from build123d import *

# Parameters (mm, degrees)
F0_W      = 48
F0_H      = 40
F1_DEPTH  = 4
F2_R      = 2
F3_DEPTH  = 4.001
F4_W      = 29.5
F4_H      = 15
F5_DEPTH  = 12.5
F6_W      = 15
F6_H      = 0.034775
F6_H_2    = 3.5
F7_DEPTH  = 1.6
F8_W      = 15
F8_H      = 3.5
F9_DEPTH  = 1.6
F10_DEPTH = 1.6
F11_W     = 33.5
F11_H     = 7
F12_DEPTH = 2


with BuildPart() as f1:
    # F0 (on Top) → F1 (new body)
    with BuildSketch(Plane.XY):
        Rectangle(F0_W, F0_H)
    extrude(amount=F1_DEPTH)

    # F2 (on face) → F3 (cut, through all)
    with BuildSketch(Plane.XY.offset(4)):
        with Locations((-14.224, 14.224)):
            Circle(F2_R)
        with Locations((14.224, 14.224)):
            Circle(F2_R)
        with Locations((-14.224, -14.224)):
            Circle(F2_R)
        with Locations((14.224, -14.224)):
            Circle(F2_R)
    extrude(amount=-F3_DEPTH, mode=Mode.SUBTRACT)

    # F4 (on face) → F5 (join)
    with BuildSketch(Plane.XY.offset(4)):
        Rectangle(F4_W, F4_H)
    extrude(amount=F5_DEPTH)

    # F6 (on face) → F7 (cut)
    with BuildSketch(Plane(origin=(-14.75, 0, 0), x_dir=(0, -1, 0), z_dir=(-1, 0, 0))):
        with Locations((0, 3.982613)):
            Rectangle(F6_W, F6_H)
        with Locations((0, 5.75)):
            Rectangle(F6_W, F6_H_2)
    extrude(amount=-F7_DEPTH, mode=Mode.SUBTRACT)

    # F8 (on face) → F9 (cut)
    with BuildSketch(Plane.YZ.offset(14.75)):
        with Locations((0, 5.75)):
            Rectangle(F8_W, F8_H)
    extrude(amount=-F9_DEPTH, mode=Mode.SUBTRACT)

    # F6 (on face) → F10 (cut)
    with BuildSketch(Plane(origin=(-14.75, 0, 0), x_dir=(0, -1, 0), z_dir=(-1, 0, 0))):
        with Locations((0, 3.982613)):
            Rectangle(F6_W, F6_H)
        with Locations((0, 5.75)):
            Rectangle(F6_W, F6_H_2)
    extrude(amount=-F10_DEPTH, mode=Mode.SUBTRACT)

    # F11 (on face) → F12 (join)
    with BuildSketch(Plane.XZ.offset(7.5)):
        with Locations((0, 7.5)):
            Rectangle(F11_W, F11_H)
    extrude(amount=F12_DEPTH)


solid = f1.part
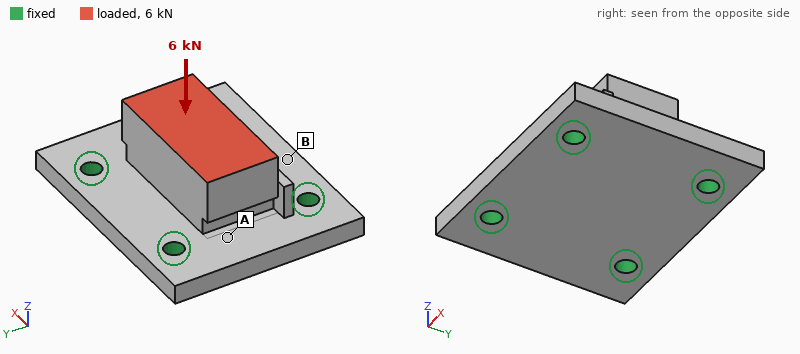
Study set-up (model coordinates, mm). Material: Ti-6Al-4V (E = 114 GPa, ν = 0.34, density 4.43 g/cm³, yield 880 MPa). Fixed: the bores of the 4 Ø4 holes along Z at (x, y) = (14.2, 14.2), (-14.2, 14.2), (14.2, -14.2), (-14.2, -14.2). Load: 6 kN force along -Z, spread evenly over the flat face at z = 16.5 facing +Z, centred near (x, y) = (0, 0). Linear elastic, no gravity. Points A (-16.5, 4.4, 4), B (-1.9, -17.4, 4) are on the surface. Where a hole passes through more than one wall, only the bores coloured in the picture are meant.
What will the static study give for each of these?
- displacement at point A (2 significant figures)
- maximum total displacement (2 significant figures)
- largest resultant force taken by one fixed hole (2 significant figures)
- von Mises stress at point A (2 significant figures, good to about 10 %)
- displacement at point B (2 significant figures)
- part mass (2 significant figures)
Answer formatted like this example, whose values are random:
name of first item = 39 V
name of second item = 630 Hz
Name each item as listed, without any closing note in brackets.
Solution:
displacement at point A = 11 µm
maximum total displacement = 20 µm
largest resultant force taken by one fixed hole = 1.6 kN
von Mises stress at point A = 40 MPa
displacement at point B = 4.0 µm
part mass = 59 g
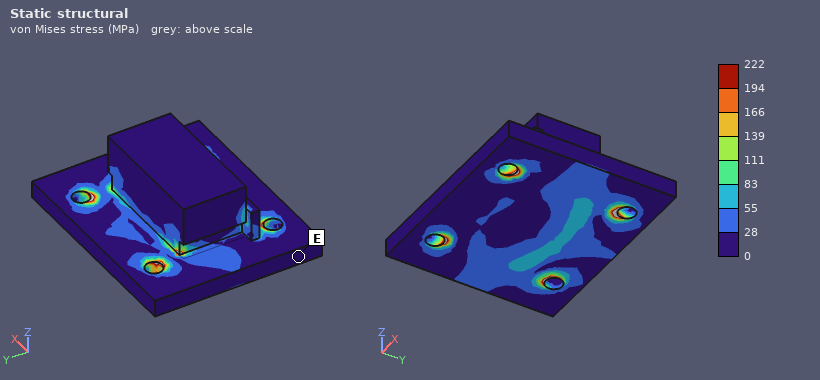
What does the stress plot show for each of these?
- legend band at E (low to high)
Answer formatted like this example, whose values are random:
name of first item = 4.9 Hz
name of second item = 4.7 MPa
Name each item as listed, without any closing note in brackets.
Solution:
legend band at E = 0 to 28 MPa
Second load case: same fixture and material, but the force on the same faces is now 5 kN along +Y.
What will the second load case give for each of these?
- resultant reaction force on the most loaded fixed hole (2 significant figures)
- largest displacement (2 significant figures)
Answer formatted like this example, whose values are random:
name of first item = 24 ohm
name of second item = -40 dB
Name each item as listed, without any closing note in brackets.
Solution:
resultant reaction force on the most loaded fixed hole = 2.1 kN
largest displacement = 32 µm
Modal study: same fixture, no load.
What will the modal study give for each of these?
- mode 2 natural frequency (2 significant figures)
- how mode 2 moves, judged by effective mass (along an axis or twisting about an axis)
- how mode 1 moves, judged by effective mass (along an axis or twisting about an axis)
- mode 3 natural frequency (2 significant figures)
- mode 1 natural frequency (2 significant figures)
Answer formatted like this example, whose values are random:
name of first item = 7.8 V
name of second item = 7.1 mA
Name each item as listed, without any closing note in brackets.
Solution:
mode 2 natural frequency = 18 kHz
how mode 2 moves, judged by effective mass = along X
how mode 1 moves, judged by effective mass = along Z
mode 3 natural frequency = 20 kHz
mode 1 natural frequency = 15 kHz
